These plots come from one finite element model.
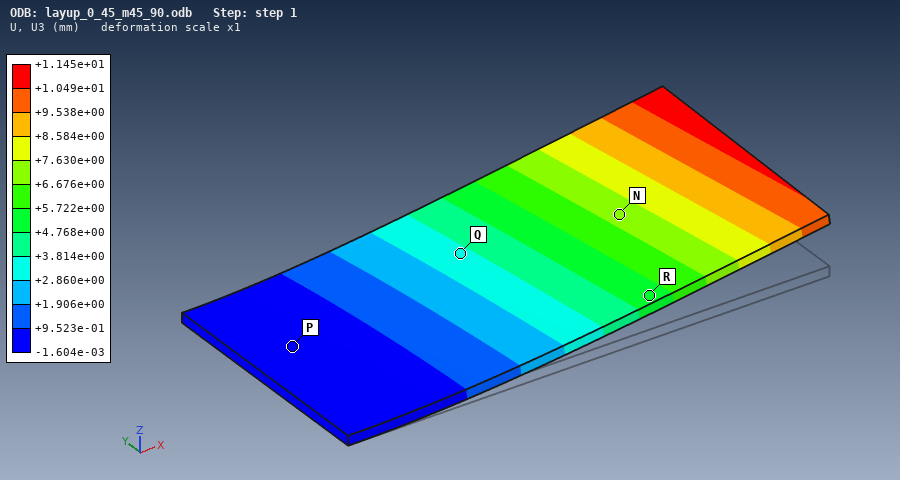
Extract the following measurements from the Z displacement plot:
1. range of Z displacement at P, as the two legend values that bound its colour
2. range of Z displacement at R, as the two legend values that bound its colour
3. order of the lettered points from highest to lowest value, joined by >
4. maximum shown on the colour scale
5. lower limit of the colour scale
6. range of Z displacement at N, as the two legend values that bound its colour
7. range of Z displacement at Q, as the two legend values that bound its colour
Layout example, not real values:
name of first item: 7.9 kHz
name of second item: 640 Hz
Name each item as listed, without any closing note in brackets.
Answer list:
range of Z displacement at P, as the two legend values that bound its colour: -1.604e-03 to +9.523e-01 mm
range of Z displacement at R, as the two legend values that bound its colour: +4.768e+00 to +5.722e+00 mm
order of the lettered points from highest to lowest value, joined by >: N > R > Q > P
maximum shown on the colour scale: +1.145e+01 mm
lower limit of the colour scale: -1.604e-03 mm
range of Z displacement at N, as the two legend values that bound its colour: +6.676e+00 to +7.630e+00 mm
range of Z displacement at Q, as the two legend values that bound its colour: +2.860e+00 to +3.814e+00 mm
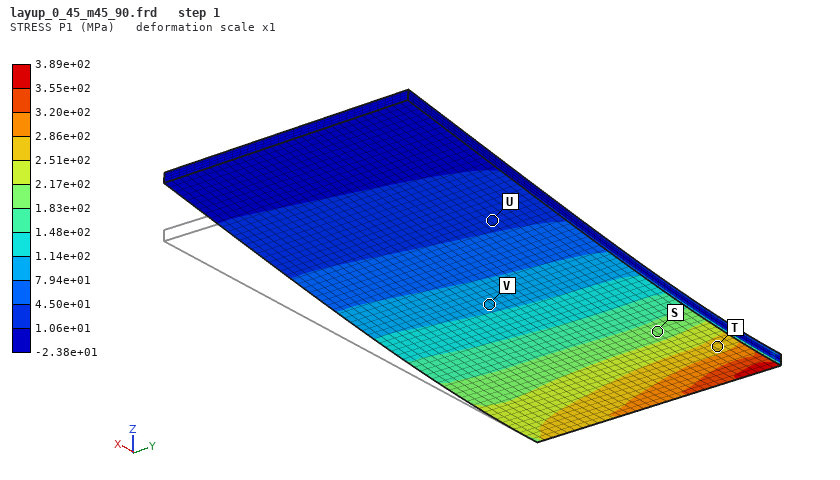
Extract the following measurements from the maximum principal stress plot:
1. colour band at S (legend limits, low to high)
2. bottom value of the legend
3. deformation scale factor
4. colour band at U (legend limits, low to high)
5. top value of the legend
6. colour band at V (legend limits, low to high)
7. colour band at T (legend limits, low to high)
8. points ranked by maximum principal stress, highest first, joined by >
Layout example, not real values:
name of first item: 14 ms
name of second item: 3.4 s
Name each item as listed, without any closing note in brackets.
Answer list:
colour band at S: 1.83e+02 to 2.17e+02 MPa
bottom value of the legend: -2.38e+01 MPa
deformation scale factor: 1
colour band at U: 1.06e+01 to 4.50e+01 MPa
top value of the legend: 3.89e+02 MPa
colour band at V: 7.94e+01 to 1.14e+02 MPa
colour band at T: 2.51e+02 to 2.86e+02 MPa
points ranked by maximum principal stress, highest first, joined by >: T > S > V > U
